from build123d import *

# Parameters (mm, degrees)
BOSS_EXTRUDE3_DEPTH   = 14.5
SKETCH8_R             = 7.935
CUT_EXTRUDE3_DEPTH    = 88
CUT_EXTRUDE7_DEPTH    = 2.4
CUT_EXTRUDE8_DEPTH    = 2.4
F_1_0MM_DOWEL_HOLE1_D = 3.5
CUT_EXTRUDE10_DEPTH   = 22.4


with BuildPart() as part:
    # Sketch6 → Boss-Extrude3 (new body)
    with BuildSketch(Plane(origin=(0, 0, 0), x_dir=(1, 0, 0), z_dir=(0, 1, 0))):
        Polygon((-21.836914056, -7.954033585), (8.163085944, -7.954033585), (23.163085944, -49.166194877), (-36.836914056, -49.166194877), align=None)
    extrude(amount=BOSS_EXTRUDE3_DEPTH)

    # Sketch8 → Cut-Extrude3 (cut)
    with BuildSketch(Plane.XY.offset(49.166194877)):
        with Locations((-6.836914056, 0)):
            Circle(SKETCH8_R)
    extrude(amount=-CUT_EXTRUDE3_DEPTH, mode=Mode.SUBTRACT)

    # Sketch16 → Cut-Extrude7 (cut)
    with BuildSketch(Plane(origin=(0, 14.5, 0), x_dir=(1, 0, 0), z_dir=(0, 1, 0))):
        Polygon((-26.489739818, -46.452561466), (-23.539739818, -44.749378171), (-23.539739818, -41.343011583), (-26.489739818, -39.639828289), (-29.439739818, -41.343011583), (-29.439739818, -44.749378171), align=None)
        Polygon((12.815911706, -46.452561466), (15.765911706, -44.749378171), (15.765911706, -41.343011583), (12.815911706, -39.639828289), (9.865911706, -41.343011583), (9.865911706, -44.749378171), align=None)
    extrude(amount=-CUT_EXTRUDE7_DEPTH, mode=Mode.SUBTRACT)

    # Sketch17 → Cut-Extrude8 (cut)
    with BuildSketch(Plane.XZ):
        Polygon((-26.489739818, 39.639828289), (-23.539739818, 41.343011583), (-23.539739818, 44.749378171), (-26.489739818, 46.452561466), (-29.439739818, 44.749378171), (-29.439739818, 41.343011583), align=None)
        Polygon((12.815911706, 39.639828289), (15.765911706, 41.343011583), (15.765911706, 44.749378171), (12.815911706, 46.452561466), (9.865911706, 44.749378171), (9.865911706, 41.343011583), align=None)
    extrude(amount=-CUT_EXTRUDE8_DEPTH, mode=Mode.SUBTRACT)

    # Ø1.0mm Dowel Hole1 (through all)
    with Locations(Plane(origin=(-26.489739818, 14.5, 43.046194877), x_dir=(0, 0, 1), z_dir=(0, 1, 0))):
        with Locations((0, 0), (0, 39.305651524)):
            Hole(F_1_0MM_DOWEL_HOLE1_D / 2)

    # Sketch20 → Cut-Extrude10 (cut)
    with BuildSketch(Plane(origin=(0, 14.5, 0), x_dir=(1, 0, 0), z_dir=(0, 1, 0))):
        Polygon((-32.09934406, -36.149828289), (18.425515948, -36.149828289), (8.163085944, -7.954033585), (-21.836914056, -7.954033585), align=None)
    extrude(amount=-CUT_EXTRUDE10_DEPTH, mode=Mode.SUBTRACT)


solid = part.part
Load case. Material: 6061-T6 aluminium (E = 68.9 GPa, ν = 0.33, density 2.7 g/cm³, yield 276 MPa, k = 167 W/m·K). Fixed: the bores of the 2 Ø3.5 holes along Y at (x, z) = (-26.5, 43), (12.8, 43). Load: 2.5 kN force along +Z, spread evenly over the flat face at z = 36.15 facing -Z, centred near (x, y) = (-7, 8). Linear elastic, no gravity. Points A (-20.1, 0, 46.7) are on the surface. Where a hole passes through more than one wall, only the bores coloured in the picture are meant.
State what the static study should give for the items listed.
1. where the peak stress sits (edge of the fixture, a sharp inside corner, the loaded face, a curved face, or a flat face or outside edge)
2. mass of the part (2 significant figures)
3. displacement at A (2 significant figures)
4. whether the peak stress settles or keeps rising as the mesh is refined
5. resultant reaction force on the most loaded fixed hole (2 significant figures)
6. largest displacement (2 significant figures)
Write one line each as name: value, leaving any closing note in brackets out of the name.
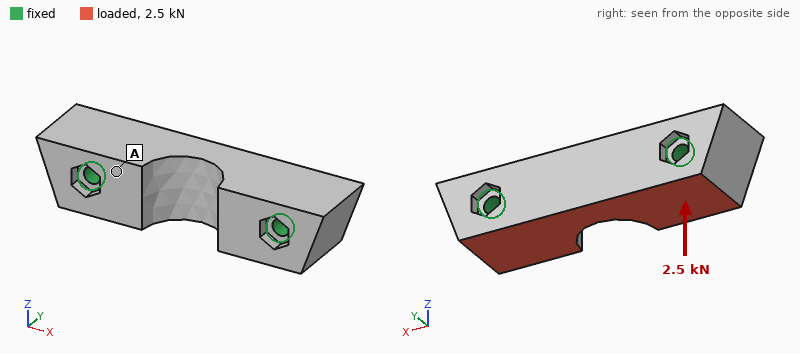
where the peak stress sits: edge of the fixture
mass of the part: 23 g
displacement at A: 3.0 µm
whether the peak stress settles or keeps rising as the mesh is refined: keeps rising
resultant reaction force on the most loaded fixed hole: 1.3 kN
largest displacement: 8.3 µm
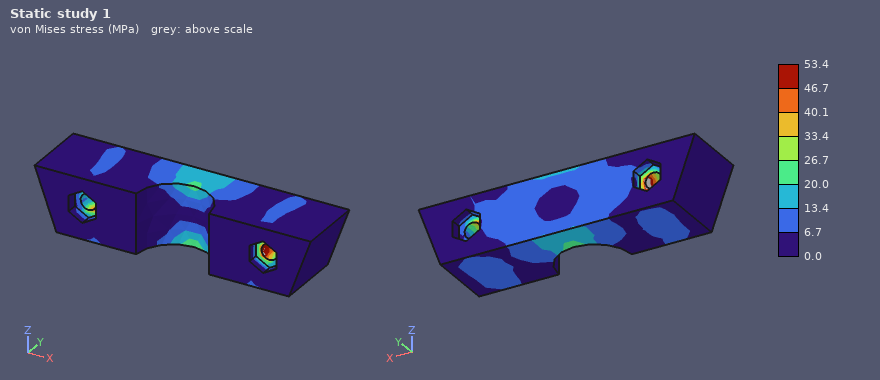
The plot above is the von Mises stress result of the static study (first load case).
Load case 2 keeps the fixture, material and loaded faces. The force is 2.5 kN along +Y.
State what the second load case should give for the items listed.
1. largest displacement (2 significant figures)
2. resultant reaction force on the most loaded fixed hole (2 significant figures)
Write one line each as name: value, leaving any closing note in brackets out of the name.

largest displacement: 13 µm
resultant reaction force on the most loaded fixed hole: 1.3 kN
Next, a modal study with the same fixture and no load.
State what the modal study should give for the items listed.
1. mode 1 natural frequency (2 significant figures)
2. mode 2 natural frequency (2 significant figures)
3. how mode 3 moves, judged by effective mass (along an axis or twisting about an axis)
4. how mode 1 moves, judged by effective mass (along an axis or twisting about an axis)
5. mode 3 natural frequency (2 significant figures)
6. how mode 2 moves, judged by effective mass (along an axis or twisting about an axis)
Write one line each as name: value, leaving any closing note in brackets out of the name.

mode 1 natural frequency: 21 kHz
mode 2 natural frequency: 25 kHz
how mode 3 moves, judged by effective mass: twisting about X
how mode 1 moves, judged by effective mass: along Z
mode 3 natural frequency: 36 kHz
how mode 2 moves, judged by effective mass: along Y
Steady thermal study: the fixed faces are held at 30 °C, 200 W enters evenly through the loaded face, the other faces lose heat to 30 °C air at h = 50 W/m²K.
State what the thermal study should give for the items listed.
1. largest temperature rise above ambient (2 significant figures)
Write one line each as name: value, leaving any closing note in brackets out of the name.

largest temperature rise above ambient: 36 K
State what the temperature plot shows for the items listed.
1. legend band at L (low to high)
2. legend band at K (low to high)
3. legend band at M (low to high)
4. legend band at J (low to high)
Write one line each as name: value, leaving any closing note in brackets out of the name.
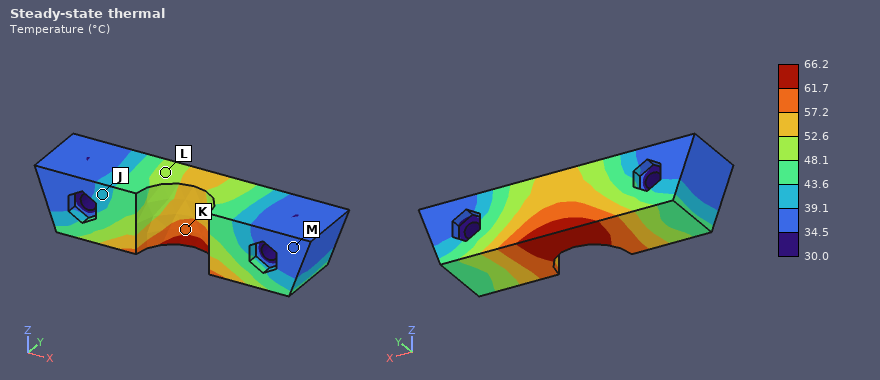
legend band at L: 48.1 to 52.6 °C
legend band at K: 57.2 to 61.7 °C
legend band at M: 34.5 to 39.1 °C
legend band at J: 39.1 to 43.6 °C
